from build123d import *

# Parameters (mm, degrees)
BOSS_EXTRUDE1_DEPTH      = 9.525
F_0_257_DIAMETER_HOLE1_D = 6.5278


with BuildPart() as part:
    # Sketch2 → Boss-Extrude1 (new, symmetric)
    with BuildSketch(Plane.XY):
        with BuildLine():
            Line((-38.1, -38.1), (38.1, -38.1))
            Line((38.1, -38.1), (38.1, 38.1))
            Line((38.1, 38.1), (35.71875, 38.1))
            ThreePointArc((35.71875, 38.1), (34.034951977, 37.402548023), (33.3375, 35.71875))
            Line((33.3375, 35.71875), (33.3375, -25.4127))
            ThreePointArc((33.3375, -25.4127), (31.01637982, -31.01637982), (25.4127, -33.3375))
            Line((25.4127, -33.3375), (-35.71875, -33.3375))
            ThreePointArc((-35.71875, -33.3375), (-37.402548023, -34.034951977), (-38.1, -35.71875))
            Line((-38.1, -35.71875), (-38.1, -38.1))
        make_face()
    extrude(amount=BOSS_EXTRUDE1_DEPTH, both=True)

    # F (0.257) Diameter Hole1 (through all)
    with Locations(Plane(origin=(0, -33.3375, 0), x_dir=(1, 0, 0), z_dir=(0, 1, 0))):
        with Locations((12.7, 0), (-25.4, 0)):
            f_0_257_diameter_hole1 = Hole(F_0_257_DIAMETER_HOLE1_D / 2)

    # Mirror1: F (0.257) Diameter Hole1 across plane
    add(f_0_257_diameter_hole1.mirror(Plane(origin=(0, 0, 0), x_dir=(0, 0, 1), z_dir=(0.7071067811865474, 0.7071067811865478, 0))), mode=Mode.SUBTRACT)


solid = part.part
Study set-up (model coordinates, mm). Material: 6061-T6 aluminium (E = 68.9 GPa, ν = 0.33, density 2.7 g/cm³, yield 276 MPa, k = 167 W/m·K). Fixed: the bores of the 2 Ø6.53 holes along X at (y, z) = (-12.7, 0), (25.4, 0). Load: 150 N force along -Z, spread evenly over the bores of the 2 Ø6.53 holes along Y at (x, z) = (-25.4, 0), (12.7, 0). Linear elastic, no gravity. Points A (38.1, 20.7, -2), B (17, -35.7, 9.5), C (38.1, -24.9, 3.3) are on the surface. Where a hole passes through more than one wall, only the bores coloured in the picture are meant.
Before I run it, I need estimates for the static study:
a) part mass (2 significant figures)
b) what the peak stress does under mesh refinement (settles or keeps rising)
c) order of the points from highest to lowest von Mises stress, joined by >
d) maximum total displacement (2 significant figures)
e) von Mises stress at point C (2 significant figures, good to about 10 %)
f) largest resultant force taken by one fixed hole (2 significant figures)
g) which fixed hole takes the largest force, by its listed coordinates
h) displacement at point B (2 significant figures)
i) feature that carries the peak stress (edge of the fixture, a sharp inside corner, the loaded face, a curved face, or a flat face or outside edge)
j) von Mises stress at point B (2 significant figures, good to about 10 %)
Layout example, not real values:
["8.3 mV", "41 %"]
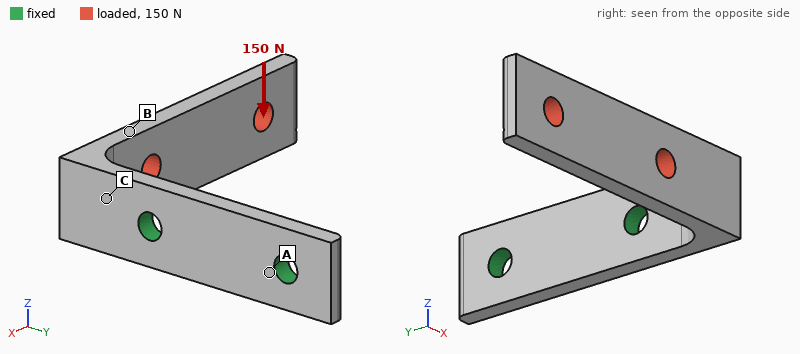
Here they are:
["35 g", "keeps rising", "C > B > A", "0.45 mm", "55 MPa", "190 N", "(-12.7, 0)", "0.12 mm", "edge of the fixture", "14 MPa"]
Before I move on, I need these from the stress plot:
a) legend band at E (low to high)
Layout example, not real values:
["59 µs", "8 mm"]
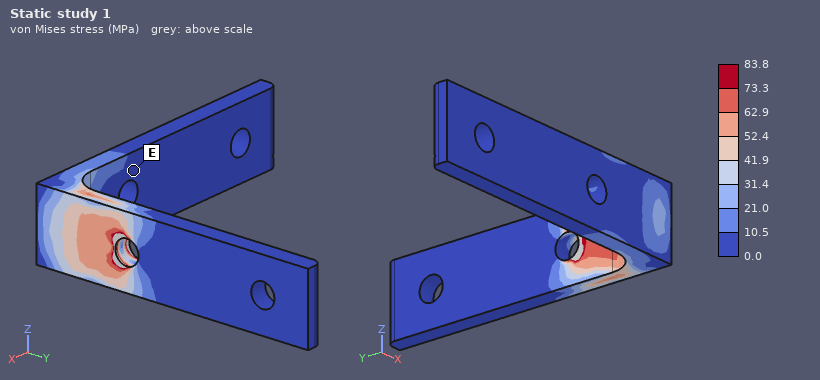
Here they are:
["0.0 to 10.5 MPa"]
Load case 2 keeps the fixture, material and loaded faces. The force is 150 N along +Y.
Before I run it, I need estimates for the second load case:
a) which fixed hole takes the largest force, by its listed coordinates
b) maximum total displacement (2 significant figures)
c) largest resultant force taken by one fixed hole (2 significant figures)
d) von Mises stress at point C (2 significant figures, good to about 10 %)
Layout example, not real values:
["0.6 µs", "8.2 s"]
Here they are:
["(-12.7, 0)", "1.2 mm", "140 N", "76 MPa"]
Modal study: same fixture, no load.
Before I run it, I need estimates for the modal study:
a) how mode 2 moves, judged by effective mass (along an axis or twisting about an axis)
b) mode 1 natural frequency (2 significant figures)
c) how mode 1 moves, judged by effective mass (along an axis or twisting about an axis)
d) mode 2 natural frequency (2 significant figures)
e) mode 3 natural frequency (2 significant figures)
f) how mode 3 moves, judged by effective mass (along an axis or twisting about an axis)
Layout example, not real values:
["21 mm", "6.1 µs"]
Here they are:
["along Z", "560 Hz", "along Y", "920 Hz", "2600 Hz", "along X"]
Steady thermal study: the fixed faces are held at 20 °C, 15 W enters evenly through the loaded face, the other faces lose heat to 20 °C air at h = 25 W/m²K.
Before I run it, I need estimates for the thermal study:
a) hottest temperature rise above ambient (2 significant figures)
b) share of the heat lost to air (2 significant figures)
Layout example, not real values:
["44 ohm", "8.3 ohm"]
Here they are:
["49 K", "22 %"]
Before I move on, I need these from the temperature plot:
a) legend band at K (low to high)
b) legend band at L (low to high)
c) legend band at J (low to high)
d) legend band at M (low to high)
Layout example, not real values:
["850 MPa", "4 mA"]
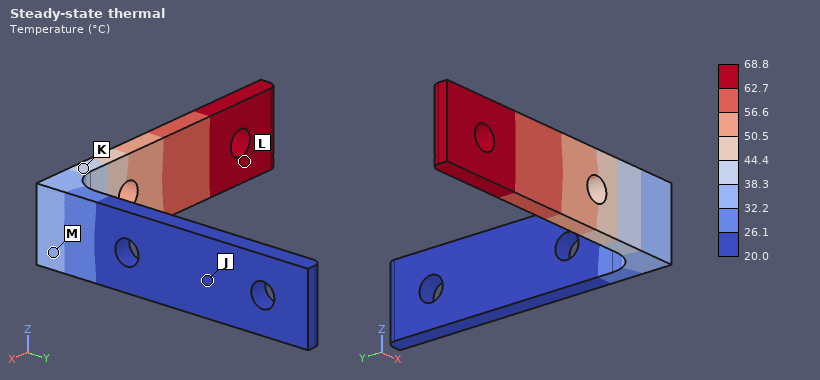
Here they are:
["38.3 to 44.4 °C", "62.7 to 68.8 °C", "20.0 to 26.1 °C", "32.2 to 38.3 °C"]
